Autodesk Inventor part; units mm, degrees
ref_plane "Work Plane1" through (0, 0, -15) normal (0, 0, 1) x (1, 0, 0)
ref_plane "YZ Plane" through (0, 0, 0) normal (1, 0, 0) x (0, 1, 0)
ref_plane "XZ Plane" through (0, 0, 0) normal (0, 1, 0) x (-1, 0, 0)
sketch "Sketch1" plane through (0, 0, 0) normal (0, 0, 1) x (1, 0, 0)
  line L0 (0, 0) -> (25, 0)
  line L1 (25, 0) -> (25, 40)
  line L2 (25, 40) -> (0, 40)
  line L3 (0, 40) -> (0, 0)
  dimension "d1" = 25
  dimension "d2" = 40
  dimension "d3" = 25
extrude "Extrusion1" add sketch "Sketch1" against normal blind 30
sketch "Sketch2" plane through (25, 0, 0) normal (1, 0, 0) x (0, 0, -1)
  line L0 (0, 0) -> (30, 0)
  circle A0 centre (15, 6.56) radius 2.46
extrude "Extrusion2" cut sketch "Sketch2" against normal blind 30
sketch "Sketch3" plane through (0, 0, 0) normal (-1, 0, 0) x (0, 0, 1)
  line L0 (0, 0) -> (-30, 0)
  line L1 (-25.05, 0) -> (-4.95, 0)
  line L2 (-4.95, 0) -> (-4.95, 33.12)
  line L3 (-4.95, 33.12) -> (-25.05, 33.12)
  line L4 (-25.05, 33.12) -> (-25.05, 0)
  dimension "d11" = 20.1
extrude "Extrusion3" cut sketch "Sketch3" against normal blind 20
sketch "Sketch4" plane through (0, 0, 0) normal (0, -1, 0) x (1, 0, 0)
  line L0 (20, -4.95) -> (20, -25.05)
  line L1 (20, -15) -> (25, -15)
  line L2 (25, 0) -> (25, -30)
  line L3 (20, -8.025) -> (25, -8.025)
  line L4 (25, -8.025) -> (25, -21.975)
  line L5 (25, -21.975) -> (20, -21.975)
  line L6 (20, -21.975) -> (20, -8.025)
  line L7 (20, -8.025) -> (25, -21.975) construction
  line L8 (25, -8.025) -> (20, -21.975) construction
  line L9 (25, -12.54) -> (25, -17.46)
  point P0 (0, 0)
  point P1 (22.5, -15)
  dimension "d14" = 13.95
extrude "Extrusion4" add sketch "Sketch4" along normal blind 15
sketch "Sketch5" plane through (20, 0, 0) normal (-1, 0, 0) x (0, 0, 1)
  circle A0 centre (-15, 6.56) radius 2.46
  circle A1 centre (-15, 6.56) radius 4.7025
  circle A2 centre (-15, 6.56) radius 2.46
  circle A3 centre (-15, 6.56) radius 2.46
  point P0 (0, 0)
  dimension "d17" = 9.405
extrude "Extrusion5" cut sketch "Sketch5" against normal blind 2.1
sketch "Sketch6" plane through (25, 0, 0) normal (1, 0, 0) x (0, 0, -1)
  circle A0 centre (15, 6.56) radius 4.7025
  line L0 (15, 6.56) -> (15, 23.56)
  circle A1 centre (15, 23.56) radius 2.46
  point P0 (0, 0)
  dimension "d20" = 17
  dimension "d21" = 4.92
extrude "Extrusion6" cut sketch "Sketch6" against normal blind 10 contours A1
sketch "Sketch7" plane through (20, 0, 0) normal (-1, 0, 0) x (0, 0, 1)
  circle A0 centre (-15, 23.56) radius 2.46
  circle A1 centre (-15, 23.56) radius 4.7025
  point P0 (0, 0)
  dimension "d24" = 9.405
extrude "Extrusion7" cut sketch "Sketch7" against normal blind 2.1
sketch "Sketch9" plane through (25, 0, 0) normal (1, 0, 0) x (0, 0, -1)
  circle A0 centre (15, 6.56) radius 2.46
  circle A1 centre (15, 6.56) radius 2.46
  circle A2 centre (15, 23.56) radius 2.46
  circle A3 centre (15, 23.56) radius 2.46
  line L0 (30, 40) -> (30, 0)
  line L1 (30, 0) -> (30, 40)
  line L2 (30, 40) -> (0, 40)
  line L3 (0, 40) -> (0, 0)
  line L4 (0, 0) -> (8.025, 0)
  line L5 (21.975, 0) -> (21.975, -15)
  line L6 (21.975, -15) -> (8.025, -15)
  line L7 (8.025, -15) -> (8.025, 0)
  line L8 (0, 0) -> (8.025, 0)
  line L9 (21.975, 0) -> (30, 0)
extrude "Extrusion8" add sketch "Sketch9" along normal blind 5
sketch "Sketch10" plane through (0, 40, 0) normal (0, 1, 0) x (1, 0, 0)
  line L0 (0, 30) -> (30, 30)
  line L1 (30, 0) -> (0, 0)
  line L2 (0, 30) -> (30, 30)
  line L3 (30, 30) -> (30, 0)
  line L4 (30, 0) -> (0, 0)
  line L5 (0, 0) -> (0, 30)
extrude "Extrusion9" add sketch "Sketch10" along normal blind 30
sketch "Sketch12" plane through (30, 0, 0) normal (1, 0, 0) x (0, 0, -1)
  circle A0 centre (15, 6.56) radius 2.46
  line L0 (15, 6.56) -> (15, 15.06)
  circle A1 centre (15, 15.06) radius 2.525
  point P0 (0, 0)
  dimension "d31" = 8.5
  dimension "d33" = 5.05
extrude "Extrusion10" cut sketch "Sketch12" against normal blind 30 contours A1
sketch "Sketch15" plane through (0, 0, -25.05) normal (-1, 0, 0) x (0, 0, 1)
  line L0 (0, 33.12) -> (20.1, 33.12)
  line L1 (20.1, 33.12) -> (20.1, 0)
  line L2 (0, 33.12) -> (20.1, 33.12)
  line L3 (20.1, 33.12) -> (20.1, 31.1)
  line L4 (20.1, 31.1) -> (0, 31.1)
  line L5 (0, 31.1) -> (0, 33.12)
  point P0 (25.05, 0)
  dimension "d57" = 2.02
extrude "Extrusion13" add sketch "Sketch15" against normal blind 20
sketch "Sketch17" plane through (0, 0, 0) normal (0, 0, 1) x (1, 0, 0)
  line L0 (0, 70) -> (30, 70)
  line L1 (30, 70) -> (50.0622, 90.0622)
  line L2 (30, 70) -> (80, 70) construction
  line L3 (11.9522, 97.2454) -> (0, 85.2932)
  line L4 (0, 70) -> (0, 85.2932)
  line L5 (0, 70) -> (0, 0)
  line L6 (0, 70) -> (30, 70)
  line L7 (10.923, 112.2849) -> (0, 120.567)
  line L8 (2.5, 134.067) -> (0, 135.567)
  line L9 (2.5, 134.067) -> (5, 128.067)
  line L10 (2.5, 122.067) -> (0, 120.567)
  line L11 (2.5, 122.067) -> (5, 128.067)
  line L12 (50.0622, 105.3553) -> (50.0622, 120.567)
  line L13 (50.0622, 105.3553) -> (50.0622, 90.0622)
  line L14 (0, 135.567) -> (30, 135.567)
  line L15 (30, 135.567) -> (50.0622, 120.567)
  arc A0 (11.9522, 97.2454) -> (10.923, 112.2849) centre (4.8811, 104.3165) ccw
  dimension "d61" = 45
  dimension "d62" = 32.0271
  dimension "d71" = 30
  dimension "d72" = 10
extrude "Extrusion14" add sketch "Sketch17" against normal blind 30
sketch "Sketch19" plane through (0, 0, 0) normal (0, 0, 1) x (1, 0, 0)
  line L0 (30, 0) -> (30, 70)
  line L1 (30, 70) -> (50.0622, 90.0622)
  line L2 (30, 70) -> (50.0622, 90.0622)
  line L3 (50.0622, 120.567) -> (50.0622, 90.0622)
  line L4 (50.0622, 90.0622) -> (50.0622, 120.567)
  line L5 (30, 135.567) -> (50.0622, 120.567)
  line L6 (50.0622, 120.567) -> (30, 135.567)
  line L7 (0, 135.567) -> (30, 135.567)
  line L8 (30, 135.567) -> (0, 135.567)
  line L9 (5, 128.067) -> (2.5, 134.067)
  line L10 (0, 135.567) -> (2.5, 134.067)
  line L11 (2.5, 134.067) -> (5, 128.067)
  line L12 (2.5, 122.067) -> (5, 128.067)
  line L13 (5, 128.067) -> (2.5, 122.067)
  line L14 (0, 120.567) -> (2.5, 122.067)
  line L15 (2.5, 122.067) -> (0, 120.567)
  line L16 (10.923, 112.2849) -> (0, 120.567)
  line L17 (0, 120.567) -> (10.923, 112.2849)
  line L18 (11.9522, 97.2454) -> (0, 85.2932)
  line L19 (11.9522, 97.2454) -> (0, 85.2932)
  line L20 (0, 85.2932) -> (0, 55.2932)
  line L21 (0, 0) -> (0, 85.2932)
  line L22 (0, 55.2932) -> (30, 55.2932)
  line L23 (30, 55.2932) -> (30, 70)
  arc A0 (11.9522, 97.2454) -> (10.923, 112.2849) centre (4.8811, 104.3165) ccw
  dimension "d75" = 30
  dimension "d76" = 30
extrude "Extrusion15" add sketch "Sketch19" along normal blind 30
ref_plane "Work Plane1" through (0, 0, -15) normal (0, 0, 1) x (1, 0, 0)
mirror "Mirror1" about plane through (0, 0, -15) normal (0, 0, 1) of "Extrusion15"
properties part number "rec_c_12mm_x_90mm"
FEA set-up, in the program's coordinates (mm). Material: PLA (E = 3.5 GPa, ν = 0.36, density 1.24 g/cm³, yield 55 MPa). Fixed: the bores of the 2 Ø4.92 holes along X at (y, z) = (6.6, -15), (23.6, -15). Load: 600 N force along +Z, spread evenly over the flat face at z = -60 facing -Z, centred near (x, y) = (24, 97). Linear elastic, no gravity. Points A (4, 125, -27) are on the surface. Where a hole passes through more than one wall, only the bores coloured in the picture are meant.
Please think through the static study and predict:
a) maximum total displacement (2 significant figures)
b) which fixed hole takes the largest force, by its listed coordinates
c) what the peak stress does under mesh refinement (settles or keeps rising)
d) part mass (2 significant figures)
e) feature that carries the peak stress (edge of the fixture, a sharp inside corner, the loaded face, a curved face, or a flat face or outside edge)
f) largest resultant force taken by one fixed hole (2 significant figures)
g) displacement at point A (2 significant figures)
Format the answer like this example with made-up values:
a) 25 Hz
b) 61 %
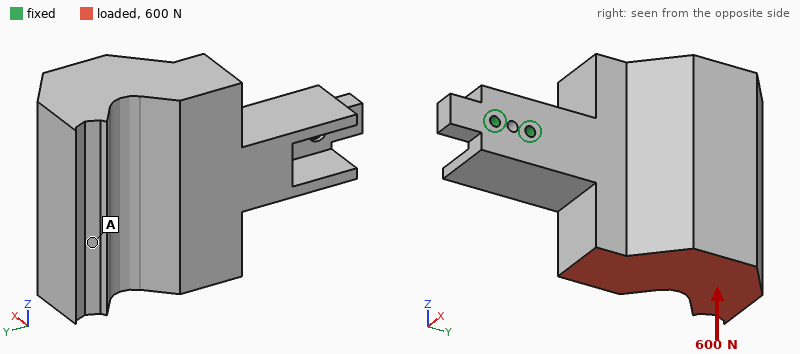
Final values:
a) 2.1 mm
b) (23.6, -15)
c) keeps rising
d) 380 g
e) edge of the fixture
f) 2.5 kN
g) 1.7 mm
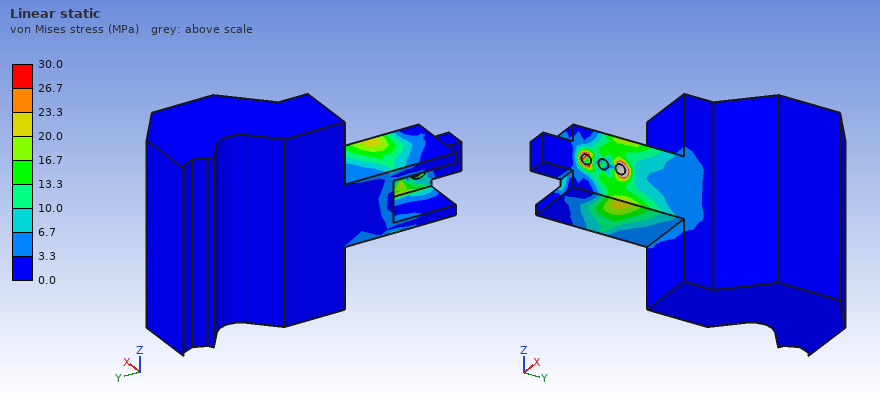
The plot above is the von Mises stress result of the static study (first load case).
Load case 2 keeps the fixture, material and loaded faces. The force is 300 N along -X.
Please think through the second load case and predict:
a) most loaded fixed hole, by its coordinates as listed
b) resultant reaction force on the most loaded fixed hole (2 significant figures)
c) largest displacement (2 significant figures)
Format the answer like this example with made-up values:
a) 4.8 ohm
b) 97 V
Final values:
a) (23.6, -15)
b) 1.2 kN
c) 2.1 mm
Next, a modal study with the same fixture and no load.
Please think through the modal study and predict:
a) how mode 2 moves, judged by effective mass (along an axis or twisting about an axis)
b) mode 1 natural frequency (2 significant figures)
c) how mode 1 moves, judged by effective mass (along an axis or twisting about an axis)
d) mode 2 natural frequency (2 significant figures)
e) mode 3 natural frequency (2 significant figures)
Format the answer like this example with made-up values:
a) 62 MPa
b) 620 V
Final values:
a) along Z
b) 150 Hz
c) along X
d) 170 Hz
e) 280 Hz
